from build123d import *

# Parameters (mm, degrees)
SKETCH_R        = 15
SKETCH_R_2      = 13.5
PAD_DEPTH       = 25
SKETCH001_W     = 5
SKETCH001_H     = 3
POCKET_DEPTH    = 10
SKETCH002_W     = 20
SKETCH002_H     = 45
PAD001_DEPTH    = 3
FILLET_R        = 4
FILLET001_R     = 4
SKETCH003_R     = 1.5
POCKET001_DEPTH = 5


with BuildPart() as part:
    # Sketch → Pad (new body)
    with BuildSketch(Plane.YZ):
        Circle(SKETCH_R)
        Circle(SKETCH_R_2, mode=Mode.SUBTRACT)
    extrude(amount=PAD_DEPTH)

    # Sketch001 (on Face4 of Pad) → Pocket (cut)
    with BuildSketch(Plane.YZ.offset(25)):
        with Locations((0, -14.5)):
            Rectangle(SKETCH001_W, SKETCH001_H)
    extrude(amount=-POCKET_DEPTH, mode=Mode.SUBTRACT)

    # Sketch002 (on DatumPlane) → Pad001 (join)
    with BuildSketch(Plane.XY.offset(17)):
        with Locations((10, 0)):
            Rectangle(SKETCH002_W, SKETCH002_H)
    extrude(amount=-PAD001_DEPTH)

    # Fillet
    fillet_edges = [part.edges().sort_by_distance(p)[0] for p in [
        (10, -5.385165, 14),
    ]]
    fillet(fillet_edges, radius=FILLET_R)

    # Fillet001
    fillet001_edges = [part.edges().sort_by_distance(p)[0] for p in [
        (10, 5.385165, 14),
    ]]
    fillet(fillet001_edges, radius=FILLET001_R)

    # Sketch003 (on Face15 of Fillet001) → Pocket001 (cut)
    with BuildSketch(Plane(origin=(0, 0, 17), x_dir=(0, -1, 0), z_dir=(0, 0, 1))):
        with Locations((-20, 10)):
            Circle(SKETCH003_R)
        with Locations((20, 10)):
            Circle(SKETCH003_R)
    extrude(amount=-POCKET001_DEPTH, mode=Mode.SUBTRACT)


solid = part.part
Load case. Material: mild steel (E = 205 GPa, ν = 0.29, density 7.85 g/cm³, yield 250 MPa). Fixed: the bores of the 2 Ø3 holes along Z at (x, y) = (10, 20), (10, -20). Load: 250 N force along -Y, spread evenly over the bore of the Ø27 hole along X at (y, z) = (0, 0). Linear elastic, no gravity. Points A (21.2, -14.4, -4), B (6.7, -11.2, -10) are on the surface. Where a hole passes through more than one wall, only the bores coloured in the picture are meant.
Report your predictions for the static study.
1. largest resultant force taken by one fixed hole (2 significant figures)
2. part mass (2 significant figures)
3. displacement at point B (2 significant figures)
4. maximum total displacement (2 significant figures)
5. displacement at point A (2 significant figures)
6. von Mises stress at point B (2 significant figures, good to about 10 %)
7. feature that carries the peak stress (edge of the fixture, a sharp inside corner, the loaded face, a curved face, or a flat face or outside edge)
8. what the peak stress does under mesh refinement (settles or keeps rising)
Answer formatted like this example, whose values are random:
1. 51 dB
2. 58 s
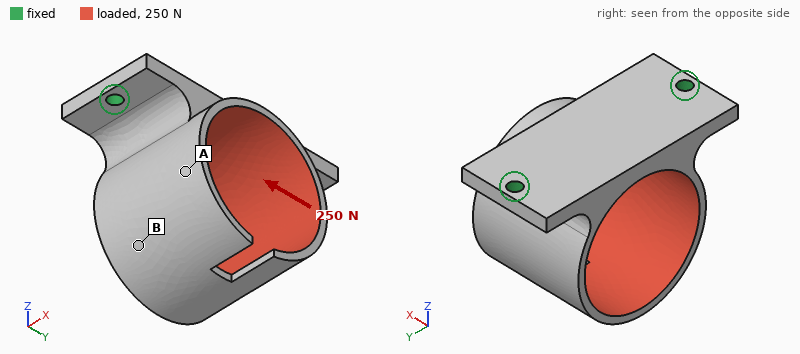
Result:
1. 170 N
2. 51 g
3. 39 µm
4. 44 µm
5. 28 µm
6. 30 MPa
7. a sharp inside corner
8. keeps rising
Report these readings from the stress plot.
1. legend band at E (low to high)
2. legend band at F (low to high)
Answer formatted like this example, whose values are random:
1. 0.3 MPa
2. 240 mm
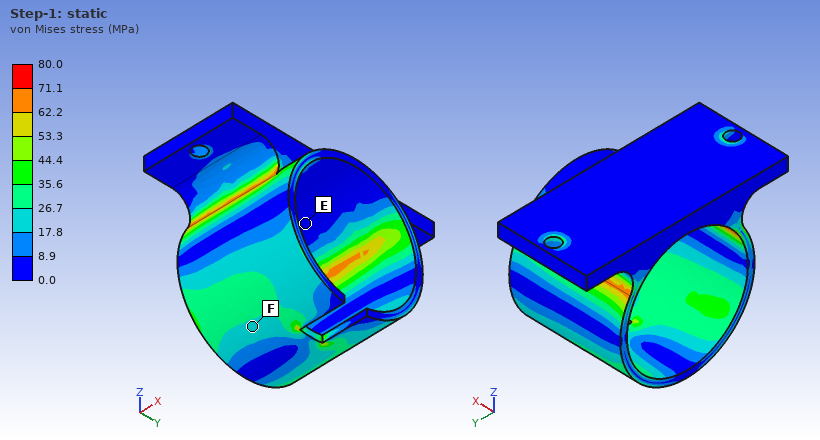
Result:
1. 0.0 to 8.9 MPa
2. 17.8 to 26.7 MPa
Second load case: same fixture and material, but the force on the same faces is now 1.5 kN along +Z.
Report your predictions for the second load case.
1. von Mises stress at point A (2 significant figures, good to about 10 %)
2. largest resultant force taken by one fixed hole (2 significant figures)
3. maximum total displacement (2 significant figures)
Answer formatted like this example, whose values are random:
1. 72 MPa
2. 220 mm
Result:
1. 45 MPa
2. 850 N
3. 62 µm
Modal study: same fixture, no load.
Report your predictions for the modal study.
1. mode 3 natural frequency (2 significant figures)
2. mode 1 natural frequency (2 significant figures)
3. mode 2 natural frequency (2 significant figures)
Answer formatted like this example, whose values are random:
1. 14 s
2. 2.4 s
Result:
1. 6400 Hz
2. 2700 Hz
3. 2700 Hz
